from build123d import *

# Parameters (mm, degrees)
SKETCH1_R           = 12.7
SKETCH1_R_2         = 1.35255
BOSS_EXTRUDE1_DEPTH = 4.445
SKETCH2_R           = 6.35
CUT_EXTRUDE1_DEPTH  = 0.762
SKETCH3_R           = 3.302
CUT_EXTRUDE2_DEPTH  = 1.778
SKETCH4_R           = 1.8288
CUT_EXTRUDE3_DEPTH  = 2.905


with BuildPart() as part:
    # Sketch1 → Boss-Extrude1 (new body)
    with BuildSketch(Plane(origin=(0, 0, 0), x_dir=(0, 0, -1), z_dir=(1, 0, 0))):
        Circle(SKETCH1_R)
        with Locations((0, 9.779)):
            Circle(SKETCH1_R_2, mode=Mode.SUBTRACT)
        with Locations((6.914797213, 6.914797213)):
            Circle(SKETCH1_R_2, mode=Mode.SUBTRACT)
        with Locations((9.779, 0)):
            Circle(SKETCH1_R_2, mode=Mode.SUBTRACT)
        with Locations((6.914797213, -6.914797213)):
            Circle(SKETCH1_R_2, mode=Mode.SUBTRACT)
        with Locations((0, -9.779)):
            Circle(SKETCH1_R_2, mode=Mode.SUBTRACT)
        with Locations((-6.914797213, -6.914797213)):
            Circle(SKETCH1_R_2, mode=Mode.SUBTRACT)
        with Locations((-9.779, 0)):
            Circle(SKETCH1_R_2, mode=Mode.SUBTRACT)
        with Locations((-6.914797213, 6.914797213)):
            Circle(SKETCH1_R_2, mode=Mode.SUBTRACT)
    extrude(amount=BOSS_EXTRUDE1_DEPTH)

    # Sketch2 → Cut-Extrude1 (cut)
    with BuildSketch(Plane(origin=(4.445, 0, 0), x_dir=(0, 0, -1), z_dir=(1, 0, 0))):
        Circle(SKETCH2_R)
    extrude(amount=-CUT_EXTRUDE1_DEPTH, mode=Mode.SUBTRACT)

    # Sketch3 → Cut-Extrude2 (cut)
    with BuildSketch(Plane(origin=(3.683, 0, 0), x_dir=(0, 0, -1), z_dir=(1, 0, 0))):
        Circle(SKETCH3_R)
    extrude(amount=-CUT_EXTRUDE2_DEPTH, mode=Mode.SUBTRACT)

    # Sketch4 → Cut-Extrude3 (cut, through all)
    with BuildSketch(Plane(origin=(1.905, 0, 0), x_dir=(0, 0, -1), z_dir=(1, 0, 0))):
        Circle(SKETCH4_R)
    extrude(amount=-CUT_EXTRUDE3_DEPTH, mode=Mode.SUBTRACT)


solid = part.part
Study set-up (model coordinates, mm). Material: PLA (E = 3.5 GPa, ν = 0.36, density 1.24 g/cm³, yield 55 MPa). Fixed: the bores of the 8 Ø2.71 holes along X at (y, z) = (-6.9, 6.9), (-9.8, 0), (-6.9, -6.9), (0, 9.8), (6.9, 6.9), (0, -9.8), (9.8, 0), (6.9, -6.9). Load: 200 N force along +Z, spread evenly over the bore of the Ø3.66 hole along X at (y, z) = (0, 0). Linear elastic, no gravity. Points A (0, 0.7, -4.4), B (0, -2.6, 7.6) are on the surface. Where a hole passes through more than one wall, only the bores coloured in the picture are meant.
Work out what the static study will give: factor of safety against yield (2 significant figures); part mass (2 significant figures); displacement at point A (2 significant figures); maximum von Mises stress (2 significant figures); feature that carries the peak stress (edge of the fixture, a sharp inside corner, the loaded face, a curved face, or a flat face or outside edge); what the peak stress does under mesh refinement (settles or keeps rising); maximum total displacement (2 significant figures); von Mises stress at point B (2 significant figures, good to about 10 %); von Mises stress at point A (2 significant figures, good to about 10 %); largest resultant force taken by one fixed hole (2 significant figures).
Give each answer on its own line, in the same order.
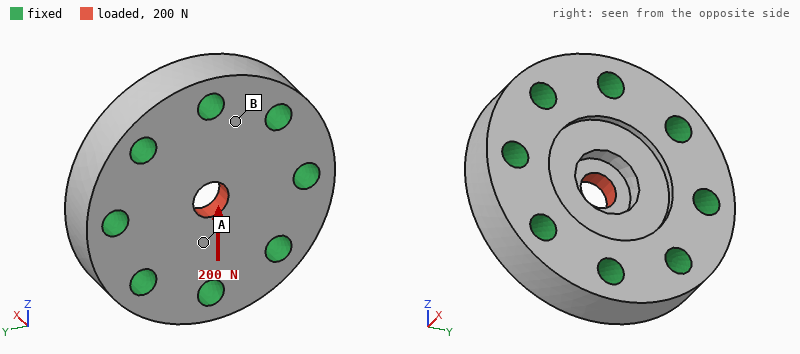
3.3
2.3 g
5.4 µm
17 MPa
the loaded face
settles
12 µm
1.6 MPa
5.7 MPa
46 N
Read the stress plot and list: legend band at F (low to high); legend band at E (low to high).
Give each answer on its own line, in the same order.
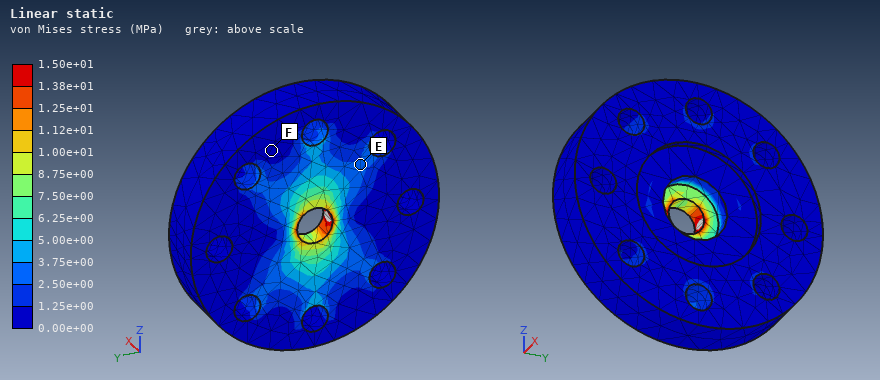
0.00e+00 to 1.25e+00 MPa
2.50e+00 to 3.75e+00 MPa
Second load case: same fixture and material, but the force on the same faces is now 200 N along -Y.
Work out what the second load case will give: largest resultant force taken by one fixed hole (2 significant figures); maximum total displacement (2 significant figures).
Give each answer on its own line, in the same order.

46 N
12 µm
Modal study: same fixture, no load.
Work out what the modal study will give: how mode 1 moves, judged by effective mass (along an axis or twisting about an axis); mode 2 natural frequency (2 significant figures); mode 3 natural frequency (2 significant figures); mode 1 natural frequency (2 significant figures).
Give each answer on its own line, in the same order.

along X
43 kHz
43 kHz
32 kHz
